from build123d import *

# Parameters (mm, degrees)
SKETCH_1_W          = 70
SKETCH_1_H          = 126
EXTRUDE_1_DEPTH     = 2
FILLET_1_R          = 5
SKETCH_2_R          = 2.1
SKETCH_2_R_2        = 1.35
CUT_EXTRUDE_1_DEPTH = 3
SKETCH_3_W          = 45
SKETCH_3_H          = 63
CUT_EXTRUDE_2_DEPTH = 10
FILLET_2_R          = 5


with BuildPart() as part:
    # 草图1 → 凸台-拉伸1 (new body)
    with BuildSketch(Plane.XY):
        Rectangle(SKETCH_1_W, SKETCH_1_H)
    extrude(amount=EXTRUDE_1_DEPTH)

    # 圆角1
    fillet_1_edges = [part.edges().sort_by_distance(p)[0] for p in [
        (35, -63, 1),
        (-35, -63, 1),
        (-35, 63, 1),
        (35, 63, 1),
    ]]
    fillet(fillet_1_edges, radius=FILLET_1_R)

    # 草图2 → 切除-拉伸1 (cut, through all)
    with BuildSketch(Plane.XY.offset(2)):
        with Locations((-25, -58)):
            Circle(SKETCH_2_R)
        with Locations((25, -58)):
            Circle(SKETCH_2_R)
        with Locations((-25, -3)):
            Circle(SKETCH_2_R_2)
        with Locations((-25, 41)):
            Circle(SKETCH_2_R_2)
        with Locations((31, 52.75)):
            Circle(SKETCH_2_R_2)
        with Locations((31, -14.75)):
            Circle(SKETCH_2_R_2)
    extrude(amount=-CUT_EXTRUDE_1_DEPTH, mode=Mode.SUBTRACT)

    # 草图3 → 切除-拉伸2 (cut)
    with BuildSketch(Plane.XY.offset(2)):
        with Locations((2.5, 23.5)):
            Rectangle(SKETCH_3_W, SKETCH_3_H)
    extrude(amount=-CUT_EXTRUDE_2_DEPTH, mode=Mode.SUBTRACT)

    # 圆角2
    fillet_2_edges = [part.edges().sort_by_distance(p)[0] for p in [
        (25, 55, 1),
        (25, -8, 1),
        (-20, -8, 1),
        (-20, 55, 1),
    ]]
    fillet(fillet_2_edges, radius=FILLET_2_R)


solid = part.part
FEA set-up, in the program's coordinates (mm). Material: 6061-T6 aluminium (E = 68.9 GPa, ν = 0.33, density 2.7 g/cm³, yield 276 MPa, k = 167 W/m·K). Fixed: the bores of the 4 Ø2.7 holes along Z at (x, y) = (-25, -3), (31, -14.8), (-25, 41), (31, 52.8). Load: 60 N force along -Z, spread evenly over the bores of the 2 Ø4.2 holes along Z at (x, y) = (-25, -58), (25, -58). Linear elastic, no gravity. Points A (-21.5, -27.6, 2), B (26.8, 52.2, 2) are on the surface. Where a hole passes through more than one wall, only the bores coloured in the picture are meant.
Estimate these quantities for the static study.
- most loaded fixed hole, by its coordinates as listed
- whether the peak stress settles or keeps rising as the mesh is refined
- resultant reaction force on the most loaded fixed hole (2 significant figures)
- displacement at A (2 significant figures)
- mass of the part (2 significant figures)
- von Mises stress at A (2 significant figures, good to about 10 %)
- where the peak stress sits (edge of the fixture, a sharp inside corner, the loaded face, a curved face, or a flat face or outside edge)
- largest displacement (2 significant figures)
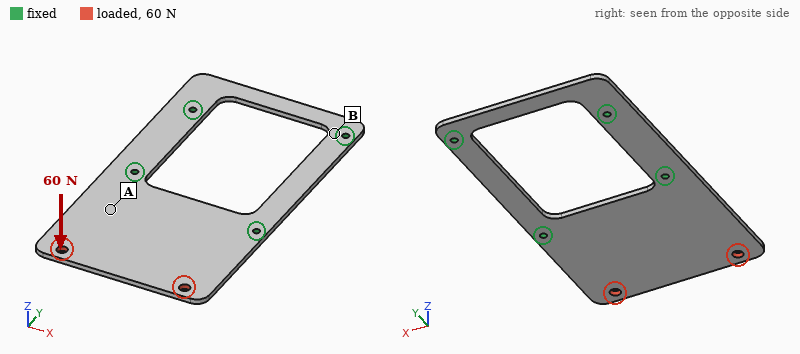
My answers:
(31, -14.8)
keeps rising
40 N
0.36 mm
32 g
33 MPa
edge of the fixture
1.4 mm
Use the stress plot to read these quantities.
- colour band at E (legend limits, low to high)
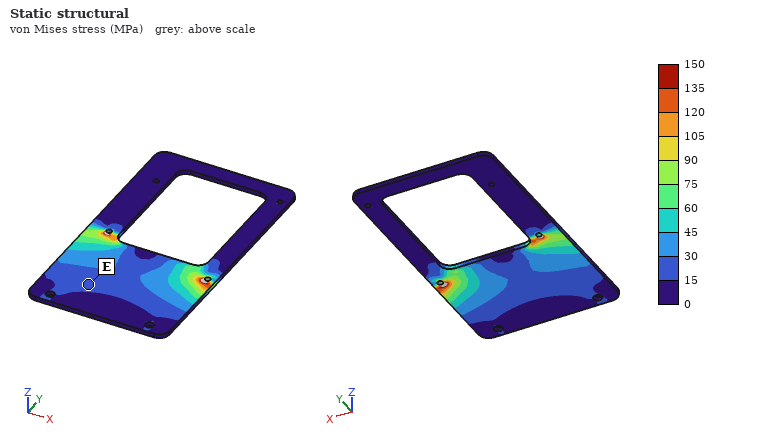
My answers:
15 to 30 MPa
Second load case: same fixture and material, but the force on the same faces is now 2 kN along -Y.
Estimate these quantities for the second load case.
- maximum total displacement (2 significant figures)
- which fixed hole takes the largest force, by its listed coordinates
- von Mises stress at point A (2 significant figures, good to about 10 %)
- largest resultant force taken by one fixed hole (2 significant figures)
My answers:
28 µm
(-25, -3)
20 MPa
1.0 kN
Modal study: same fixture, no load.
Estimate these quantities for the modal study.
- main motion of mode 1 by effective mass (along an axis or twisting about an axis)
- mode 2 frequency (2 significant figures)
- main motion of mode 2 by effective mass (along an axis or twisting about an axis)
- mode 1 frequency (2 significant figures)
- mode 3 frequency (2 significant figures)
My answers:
along Z
1200 Hz
twisting about Y
440 Hz
2300 Hz
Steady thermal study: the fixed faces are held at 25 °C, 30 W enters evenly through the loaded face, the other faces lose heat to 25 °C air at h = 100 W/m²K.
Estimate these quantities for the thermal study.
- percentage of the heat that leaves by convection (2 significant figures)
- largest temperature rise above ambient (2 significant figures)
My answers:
65 %
59 K
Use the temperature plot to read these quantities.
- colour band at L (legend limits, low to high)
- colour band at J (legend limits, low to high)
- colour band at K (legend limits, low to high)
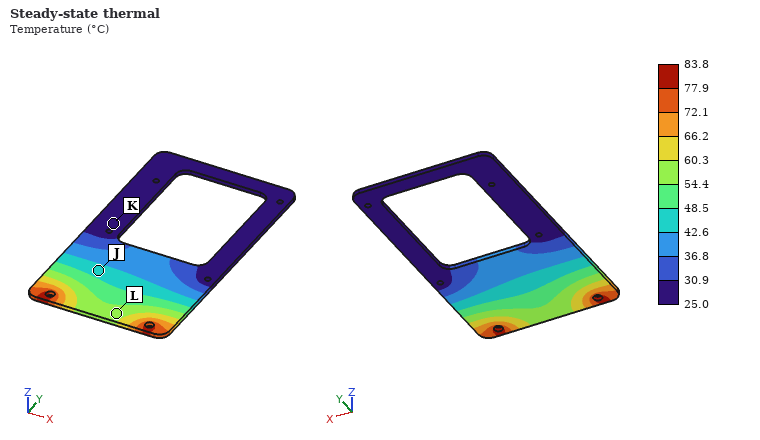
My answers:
54.4 to 60.3 °C
42.6 to 48.5 °C
25.0 to 30.9 °C
